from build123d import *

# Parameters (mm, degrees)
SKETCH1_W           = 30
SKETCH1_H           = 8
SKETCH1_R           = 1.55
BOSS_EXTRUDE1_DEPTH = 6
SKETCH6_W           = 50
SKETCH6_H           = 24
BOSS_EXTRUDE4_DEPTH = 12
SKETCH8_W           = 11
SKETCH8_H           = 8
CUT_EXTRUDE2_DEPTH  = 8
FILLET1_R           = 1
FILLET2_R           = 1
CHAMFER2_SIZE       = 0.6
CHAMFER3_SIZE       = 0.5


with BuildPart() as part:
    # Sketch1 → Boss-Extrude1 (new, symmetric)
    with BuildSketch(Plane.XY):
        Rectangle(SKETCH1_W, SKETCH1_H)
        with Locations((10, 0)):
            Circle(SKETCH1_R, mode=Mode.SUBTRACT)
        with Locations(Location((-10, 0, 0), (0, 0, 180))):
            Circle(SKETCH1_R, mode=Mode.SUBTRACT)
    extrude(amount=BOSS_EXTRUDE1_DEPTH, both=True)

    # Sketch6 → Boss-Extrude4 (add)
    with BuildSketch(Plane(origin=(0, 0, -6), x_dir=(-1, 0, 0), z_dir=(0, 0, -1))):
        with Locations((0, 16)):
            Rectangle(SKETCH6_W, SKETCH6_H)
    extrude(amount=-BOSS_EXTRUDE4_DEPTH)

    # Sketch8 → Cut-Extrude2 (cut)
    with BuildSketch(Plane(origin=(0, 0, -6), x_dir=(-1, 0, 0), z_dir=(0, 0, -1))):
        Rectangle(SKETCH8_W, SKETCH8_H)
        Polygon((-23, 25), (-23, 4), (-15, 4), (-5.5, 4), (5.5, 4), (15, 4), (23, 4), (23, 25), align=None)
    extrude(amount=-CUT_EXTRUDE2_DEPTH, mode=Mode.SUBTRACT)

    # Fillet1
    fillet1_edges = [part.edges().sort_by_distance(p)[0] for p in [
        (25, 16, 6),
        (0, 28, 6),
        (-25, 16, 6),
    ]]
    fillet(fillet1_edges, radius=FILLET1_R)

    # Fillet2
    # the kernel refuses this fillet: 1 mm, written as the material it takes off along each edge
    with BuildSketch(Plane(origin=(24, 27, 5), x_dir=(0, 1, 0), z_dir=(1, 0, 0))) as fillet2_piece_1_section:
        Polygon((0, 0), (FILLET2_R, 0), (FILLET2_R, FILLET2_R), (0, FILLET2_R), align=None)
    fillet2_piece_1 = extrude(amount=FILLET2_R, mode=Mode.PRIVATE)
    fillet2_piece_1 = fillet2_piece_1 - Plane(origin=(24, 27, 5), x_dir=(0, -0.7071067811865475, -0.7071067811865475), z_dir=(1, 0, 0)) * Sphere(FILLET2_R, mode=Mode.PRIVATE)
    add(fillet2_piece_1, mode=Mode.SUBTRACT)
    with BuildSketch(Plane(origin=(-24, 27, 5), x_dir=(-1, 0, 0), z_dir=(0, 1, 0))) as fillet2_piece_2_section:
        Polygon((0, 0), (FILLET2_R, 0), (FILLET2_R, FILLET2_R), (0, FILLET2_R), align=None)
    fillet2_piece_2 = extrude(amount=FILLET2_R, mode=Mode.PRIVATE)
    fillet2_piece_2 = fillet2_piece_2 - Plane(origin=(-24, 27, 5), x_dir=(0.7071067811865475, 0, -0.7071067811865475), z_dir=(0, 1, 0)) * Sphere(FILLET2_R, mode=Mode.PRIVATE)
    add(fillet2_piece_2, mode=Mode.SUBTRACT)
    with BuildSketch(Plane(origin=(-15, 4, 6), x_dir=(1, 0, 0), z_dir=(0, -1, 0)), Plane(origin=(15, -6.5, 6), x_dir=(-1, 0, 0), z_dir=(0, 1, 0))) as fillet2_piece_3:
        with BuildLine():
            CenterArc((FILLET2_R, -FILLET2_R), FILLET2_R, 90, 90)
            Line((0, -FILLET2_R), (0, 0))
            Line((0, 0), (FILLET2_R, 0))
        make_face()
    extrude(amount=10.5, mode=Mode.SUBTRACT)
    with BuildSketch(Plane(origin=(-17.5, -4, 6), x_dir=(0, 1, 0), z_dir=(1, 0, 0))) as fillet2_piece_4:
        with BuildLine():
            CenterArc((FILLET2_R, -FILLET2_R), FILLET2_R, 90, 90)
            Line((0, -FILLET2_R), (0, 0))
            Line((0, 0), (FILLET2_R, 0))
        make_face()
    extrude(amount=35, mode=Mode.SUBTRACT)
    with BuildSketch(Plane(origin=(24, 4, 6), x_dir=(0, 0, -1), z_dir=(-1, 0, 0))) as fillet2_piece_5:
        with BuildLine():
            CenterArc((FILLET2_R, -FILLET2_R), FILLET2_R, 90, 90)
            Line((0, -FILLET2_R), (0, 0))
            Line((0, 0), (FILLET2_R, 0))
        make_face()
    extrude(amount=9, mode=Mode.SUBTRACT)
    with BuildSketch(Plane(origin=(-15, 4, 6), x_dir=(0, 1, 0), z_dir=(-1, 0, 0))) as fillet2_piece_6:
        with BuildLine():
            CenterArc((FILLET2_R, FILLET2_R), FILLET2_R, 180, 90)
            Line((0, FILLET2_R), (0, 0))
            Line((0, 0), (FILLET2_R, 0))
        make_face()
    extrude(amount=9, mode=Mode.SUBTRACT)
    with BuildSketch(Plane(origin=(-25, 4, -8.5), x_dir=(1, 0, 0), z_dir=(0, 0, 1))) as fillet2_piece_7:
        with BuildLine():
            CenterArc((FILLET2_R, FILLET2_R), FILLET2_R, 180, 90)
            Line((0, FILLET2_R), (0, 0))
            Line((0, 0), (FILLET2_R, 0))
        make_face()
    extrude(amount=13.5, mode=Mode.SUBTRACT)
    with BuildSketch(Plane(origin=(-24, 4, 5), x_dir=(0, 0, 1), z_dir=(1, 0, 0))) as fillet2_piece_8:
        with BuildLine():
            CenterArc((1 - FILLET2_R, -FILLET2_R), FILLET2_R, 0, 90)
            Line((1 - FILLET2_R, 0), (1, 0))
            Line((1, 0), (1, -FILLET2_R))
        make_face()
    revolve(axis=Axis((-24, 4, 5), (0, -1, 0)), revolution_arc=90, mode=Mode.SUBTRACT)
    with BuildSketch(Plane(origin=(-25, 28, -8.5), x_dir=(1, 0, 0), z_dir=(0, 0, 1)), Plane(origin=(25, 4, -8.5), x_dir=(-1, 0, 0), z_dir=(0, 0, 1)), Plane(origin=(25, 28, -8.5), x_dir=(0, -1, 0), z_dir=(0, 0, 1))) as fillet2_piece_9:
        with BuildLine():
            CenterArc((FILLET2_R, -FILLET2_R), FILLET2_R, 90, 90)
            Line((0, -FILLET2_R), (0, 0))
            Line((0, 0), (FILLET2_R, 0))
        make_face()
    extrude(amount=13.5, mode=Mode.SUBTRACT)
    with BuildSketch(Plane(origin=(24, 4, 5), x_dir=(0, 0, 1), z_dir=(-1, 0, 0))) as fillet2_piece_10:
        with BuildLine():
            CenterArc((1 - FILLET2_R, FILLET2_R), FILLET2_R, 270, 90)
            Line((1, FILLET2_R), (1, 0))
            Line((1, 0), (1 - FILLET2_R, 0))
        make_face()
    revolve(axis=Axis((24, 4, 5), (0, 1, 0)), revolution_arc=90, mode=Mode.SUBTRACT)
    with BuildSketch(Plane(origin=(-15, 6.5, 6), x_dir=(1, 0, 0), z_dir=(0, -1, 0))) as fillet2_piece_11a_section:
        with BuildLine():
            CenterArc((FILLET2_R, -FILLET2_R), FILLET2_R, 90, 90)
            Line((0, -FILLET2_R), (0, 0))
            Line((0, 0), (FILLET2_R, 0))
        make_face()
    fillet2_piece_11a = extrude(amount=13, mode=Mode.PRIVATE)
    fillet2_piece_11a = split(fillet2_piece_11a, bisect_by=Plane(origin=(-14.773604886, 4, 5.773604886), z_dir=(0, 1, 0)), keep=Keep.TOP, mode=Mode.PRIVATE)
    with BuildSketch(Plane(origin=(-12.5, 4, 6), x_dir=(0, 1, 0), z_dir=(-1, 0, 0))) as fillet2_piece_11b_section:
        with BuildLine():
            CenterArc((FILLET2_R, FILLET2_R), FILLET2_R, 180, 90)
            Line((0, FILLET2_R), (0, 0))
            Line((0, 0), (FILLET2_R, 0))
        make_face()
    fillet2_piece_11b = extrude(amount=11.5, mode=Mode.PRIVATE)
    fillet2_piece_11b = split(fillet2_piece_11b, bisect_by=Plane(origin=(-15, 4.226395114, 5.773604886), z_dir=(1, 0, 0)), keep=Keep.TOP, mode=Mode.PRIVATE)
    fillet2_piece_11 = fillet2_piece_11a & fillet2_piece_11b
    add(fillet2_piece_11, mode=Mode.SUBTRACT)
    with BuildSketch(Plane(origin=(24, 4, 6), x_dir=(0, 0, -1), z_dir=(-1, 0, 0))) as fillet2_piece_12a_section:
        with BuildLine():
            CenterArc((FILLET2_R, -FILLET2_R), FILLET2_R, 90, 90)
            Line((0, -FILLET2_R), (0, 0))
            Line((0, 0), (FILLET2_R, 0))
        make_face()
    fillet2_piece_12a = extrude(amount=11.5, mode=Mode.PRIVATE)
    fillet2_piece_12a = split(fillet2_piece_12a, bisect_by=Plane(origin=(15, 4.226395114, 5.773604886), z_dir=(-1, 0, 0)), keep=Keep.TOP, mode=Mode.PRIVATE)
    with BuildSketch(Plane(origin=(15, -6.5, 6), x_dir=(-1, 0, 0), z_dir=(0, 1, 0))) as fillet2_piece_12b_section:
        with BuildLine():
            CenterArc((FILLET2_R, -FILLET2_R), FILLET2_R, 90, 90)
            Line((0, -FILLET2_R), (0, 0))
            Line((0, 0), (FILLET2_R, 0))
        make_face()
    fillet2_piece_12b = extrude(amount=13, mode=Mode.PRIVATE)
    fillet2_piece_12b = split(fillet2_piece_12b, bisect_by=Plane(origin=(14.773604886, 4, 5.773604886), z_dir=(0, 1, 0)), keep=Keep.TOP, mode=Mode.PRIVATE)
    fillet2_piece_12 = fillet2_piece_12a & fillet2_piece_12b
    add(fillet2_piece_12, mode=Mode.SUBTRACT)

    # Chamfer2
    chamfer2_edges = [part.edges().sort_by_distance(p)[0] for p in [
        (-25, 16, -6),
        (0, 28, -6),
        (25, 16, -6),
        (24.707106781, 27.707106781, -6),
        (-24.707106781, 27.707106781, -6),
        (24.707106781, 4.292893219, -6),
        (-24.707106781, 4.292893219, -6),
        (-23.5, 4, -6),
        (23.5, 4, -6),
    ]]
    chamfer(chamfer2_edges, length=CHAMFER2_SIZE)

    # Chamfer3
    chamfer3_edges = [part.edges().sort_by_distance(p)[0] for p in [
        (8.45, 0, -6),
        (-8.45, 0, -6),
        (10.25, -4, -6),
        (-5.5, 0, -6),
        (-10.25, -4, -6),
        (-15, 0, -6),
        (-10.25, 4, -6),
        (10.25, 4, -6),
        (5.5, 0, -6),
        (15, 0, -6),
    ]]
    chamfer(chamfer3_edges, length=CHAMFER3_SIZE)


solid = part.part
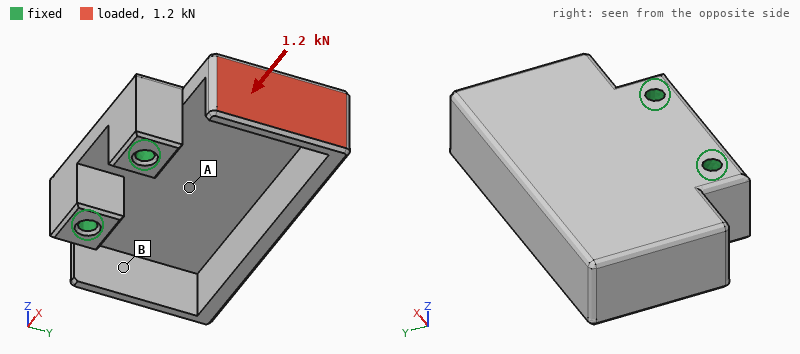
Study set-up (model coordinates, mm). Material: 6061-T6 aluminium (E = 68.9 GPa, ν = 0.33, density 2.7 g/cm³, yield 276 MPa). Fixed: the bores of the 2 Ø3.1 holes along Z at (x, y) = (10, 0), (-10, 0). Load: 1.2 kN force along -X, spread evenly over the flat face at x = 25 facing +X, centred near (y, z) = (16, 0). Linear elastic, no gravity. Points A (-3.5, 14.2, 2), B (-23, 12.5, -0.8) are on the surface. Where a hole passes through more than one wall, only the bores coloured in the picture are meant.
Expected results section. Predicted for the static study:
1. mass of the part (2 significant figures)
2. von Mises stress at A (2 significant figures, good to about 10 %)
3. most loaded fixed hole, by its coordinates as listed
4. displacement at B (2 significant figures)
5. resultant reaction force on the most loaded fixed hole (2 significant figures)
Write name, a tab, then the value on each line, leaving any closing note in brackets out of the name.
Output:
mass of the part	23 g
von Mises stress at A	36 MPa
most loaded fixed hole, by its coordinates as listed	(10, 0)
displacement at B	0.033 mm
resultant reaction force on the most loaded fixed hole	1.1 kN
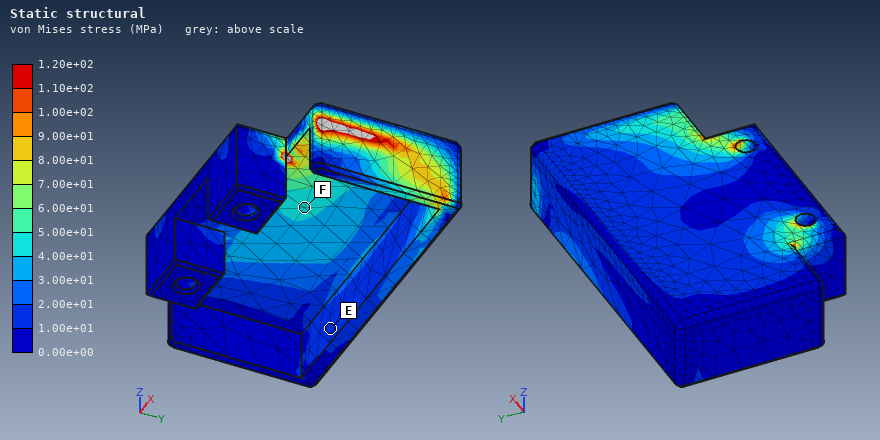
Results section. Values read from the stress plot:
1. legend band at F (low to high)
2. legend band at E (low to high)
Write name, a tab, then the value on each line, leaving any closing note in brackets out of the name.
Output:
legend band at F	4.00e+01 to 5.00e+01 MPa
legend band at E	1.00e+01 to 2.00e+01 MPa
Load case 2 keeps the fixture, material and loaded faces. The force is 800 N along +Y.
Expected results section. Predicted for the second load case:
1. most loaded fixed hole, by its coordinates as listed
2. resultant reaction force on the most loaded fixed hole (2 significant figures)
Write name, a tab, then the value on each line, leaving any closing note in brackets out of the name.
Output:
most loaded fixed hole, by its coordinates as listed	(10, 0)
resultant reaction force on the most loaded fixed hole	1.3 kN
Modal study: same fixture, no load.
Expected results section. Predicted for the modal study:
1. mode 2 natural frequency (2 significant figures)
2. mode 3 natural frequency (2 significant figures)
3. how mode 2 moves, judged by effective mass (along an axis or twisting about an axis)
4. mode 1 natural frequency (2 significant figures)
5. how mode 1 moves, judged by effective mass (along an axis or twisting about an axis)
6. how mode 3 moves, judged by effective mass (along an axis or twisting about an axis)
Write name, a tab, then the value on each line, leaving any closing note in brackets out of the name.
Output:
mode 2 natural frequency	3900 Hz
mode 3 natural frequency	9900 Hz
how mode 2 moves, judged by effective mass	twisting about Y
mode 1 natural frequency	2800 Hz
how mode 1 moves, judged by effective mass	along Z
how mode 3 moves, judged by effective mass	along X
